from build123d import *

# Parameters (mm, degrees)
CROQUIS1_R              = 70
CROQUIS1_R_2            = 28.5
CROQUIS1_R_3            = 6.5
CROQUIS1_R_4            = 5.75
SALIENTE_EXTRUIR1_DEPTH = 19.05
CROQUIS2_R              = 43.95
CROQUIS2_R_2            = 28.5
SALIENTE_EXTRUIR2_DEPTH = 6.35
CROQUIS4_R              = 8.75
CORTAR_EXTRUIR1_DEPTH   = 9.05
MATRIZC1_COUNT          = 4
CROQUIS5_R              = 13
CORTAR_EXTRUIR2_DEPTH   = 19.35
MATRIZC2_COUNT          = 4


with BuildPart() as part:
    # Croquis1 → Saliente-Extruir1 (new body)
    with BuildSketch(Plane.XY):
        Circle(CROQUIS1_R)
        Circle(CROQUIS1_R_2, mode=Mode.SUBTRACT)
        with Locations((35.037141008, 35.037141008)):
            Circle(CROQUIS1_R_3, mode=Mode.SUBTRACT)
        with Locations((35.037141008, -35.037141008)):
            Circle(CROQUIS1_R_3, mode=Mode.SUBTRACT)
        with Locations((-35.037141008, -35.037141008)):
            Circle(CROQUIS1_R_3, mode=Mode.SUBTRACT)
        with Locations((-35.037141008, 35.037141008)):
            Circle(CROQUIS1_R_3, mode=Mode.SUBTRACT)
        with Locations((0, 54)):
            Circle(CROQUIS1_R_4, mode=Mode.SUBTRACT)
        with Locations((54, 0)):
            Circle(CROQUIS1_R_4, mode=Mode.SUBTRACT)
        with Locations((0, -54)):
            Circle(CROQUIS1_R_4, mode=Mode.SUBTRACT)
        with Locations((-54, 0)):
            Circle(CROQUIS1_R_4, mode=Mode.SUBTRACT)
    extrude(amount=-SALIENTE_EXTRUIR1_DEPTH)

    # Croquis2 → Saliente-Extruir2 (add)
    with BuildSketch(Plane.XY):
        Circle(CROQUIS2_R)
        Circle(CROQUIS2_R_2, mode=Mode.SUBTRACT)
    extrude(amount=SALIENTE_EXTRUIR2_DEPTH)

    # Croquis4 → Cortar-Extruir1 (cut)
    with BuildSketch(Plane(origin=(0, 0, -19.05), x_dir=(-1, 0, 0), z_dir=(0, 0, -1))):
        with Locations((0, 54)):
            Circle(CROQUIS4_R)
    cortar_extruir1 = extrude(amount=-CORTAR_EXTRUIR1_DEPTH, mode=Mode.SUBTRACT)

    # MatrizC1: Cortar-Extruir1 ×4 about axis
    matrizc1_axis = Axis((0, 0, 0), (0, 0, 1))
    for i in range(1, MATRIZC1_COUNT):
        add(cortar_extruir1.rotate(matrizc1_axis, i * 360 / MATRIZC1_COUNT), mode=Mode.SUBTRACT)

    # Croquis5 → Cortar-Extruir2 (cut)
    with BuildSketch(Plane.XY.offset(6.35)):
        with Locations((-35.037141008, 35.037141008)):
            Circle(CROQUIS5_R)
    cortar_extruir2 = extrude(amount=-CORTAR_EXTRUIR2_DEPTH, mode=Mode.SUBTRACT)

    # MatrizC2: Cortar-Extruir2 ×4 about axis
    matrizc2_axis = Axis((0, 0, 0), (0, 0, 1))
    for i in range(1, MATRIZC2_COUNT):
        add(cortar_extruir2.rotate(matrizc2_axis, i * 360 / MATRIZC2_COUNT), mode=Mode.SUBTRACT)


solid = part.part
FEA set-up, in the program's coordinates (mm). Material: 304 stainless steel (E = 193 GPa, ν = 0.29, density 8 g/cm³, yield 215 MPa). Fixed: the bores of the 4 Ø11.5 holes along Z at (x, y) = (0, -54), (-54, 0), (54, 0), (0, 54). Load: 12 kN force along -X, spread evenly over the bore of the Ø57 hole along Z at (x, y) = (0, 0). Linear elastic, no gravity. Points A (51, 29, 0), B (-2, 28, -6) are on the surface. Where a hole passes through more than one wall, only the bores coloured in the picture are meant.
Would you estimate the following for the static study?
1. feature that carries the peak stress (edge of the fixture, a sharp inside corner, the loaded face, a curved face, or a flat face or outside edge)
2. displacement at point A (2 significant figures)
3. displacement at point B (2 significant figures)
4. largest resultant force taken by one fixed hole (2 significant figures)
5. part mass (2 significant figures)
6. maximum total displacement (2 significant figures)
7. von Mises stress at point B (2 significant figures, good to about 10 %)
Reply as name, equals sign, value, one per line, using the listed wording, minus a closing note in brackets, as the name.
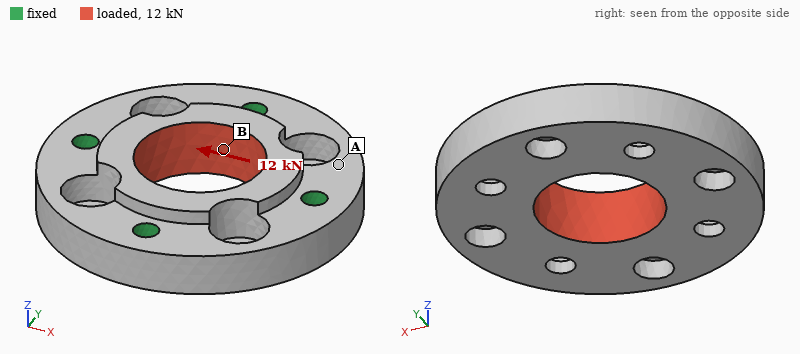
feature that carries the peak stress = edge of the fixture
displacement at point A = 0.61 µm
displacement at point B = 1.5 µm
largest resultant force taken by one fixed hole = 3.5 kN
part mass = 1.8 kg
maximum total displacement = 1.8 µm
von Mises stress at point B = 4.9 MPa
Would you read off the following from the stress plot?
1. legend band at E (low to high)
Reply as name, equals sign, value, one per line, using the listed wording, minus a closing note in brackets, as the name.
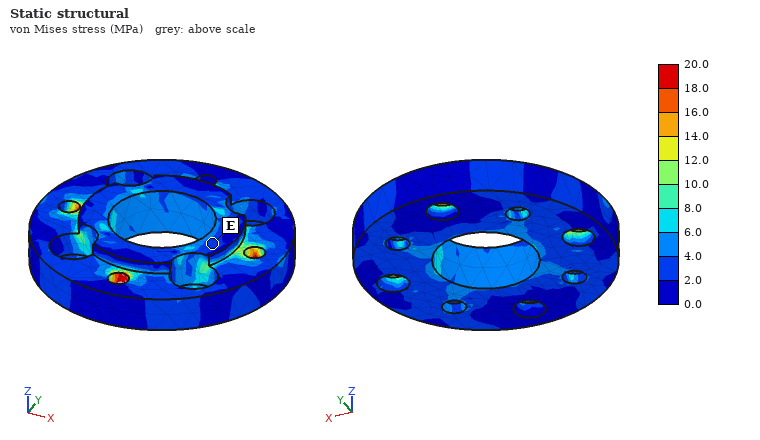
legend band at E = 2.0 to 4.0 MPa
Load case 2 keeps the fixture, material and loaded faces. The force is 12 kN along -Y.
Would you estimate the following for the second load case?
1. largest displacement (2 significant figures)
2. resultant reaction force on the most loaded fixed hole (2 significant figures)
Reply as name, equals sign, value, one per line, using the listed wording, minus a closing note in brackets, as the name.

largest displacement = 1.8 µm
resultant reaction force on the most loaded fixed hole = 3.5 kN
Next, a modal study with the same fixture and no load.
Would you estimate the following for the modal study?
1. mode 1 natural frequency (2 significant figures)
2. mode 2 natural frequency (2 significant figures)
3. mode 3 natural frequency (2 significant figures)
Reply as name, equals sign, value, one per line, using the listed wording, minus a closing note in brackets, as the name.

mode 1 natural frequency = 7000 Hz
mode 2 natural frequency = 8400 Hz
mode 3 natural frequency = 8400 Hz
